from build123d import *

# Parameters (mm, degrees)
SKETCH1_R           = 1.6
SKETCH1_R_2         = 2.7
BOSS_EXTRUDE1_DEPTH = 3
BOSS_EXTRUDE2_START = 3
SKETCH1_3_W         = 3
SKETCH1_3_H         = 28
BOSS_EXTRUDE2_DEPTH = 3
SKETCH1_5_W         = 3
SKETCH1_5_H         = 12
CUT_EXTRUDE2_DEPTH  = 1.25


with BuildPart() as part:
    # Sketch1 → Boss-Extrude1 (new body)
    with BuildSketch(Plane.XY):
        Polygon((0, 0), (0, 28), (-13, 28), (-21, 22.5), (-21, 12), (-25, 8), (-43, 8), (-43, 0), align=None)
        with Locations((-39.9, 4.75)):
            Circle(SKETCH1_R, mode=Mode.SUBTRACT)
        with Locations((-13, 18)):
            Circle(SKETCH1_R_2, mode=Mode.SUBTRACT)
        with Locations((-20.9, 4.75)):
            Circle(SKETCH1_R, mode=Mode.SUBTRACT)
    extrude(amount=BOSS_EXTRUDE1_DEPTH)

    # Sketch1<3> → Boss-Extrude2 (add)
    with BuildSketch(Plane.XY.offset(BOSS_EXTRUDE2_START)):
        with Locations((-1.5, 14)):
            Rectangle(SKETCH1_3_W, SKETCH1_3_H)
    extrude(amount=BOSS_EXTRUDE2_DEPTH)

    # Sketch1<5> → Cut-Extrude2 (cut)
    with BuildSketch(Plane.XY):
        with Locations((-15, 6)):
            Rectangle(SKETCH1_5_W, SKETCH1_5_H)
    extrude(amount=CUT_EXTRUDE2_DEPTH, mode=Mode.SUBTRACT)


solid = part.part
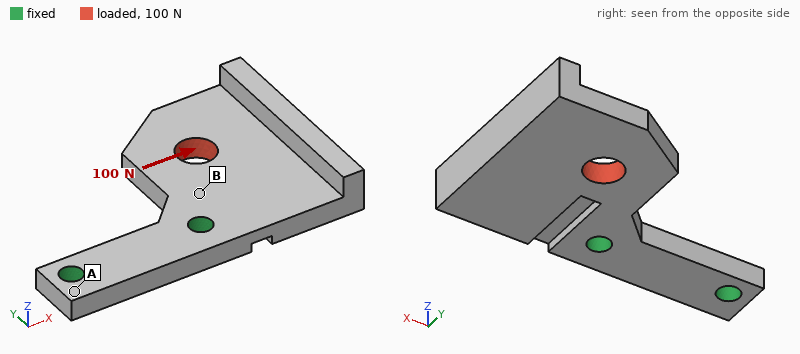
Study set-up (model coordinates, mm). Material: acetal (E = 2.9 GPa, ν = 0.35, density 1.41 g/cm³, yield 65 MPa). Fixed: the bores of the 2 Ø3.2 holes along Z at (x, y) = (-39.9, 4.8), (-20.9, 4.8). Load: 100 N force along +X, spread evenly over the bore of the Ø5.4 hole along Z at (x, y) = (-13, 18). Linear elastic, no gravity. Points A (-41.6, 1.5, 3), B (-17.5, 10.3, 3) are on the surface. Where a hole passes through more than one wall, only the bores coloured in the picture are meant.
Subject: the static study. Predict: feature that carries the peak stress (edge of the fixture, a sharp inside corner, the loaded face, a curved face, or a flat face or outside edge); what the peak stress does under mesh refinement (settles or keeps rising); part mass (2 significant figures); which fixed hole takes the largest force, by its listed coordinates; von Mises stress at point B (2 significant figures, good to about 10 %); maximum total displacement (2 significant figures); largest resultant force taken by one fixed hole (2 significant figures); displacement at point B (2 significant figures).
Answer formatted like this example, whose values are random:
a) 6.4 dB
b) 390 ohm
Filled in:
a) edge of the fixture
b) keeps rising
c) 3.3 g
d) (-20.9, 4.8)
e) 11 MPa
f) 0.50 mm
g) 100 N
h) 0.084 mm
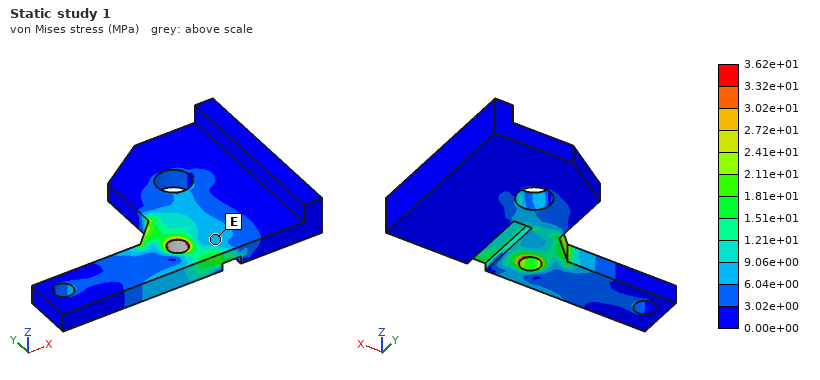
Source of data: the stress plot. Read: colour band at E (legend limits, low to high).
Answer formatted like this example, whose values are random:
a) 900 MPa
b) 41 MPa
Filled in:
a) 6.04e+00 to 9.06e+00 MPa
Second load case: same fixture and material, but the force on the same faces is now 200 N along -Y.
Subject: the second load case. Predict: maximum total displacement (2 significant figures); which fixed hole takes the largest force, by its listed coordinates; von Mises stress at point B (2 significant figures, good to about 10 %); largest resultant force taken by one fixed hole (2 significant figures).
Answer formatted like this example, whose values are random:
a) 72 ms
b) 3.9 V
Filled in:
a) 0.60 mm
b) (-20.9, 4.8)
c) 14 MPa
d) 230 N
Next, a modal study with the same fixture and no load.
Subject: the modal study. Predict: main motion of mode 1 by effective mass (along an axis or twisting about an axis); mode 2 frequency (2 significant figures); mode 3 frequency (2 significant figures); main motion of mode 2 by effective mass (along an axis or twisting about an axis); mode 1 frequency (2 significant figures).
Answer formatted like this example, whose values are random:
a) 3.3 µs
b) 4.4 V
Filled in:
a) along Z
b) 1300 Hz
c) 1600 Hz
d) twisting about X
e) 610 Hz
